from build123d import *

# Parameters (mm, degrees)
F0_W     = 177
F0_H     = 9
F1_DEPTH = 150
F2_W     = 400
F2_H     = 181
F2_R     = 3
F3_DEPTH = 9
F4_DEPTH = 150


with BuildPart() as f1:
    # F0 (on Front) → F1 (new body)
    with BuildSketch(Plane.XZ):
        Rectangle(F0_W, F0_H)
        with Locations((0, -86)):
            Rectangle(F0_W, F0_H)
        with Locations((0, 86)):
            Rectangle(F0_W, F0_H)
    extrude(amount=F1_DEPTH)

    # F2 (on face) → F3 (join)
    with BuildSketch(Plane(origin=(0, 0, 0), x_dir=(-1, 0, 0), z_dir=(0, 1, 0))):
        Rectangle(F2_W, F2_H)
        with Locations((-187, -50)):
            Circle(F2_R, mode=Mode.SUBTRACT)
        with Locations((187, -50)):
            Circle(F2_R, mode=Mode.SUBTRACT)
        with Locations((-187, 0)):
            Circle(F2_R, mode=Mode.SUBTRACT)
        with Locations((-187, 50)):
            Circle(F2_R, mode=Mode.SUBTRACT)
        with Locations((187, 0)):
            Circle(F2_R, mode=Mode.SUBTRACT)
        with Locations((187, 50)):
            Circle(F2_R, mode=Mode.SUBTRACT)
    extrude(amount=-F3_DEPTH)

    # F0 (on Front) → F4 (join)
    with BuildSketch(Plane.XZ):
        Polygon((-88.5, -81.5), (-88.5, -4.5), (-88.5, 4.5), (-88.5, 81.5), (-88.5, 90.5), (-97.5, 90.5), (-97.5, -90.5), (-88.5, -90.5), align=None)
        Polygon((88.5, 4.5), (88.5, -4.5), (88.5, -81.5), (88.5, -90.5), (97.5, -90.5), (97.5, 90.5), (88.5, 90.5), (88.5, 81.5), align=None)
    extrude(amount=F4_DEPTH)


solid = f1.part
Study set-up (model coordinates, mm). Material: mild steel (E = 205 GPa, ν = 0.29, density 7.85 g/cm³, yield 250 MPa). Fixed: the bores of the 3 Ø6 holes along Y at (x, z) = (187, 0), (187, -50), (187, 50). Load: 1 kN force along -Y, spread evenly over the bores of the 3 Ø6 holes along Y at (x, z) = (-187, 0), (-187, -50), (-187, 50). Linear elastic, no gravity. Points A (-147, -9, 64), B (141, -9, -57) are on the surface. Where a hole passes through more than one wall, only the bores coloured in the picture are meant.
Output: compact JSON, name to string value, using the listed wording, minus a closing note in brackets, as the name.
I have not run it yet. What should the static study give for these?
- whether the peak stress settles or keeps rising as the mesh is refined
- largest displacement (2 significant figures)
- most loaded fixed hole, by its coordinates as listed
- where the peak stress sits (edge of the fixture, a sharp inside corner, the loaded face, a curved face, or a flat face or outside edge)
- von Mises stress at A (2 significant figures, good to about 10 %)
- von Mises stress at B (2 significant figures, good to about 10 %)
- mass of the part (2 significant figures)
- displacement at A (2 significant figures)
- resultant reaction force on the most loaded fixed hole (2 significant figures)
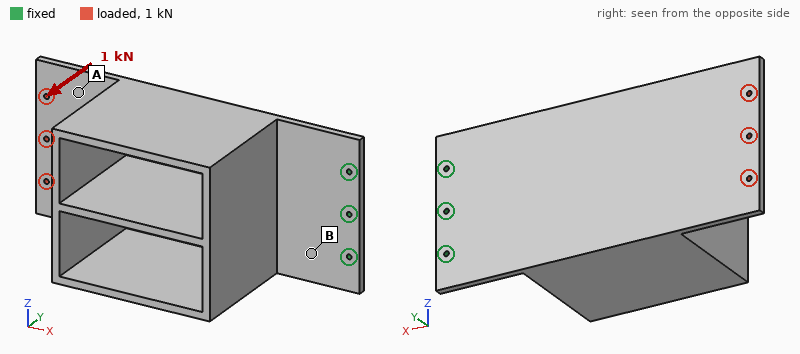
{"whether the peak stress settles or keeps rising as the mesh is refined": "keeps rising", "largest displacement": "5.2 mm", "most loaded fixed hole, by its coordinates as listed": "(187, 0)", "where the peak stress sits": "edge of the fixture", "von Mises stress at A": "16 MPa", "von Mises stress at B": "120 MPa", "mass of the part": "14 kg", "displacement at A": "4.3 mm", "resultant reaction force on the most loaded fixed hole": "820 N"}
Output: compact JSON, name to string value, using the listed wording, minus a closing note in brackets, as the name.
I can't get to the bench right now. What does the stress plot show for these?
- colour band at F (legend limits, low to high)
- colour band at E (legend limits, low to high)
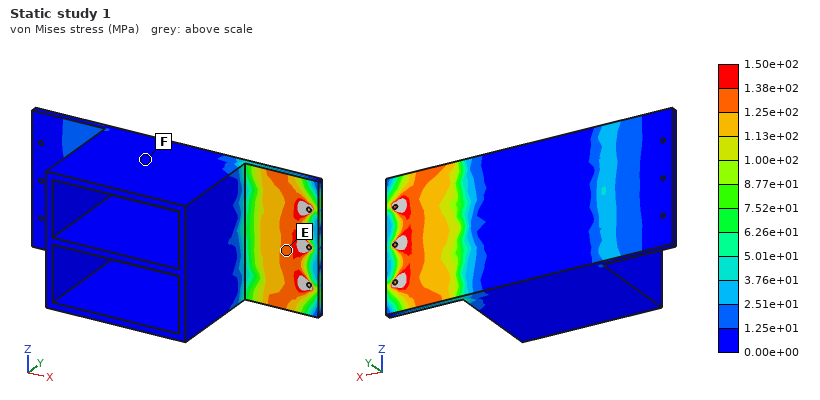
{"colour band at F": "0.00e+00 to 1.25e+01 MPa", "colour band at E": "1.25e+02 to 1.38e+02 MPa"}
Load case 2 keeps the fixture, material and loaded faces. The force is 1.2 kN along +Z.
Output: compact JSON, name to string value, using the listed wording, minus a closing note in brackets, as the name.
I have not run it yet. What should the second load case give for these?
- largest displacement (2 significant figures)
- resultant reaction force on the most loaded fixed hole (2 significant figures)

{"largest displacement": "42 µm", "resultant reaction force on the most loaded fixed hole": "4.4 kN"}
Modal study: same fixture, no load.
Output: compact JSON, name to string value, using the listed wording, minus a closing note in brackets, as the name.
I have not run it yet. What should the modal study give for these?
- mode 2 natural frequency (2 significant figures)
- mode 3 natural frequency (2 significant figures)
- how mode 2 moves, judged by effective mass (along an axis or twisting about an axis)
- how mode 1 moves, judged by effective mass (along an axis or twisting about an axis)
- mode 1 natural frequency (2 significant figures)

{"mode 2 natural frequency": "140 Hz", "mode 3 natural frequency": "390 Hz", "how mode 2 moves, judged by effective mass": "along Z", "how mode 1 moves, judged by effective mass": "along Y", "mode 1 natural frequency": "35 Hz"}
